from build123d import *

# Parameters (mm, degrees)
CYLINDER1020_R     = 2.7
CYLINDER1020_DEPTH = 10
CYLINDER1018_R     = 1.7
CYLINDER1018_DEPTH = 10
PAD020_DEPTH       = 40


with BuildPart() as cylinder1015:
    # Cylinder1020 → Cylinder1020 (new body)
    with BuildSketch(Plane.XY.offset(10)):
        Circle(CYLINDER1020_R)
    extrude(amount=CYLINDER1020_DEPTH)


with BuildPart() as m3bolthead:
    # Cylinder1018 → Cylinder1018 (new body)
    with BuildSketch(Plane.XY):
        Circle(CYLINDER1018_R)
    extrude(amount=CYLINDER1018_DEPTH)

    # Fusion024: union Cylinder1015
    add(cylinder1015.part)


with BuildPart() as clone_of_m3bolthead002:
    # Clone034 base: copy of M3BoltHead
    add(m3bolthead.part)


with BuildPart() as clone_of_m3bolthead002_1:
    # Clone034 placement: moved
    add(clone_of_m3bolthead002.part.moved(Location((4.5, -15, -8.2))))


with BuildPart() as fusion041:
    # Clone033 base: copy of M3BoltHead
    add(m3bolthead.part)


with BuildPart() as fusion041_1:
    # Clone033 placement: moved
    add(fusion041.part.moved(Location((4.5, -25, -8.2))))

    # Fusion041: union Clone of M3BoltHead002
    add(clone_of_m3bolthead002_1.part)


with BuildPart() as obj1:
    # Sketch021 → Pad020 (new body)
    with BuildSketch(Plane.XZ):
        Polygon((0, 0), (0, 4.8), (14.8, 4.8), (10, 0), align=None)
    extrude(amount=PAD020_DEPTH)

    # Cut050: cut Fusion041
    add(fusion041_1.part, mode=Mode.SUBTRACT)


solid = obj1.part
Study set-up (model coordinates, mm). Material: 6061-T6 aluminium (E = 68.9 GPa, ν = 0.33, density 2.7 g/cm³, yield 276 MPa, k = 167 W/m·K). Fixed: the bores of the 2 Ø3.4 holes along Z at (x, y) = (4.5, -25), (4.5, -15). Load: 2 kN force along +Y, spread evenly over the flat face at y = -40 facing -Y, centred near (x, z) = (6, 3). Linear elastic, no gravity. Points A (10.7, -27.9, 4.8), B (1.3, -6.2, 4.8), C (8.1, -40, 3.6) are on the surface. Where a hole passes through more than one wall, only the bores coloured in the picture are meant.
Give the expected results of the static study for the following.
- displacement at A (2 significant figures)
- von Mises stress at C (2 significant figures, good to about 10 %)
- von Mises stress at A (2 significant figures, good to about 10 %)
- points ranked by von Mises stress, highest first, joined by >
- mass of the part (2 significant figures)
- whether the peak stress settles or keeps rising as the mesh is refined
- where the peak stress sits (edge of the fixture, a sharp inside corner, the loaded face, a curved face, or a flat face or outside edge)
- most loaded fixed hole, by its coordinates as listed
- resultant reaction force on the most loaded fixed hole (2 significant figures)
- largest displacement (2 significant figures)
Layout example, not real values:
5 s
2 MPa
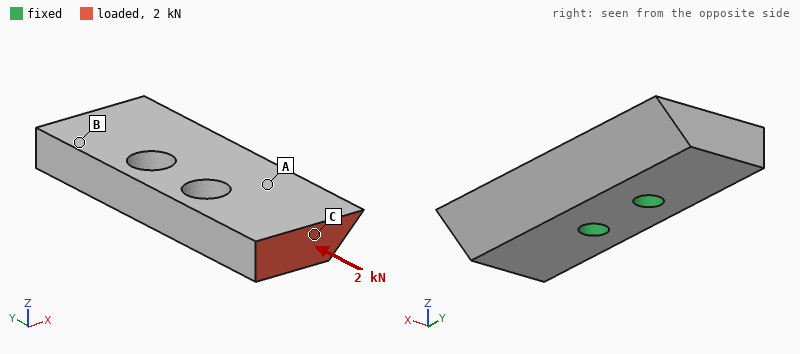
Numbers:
12 µm
33 MPa
53 MPa
A > C > B
6.0 g
keeps rising
edge of the fixture
(4.5, -25)
1.4 kN
31 µm
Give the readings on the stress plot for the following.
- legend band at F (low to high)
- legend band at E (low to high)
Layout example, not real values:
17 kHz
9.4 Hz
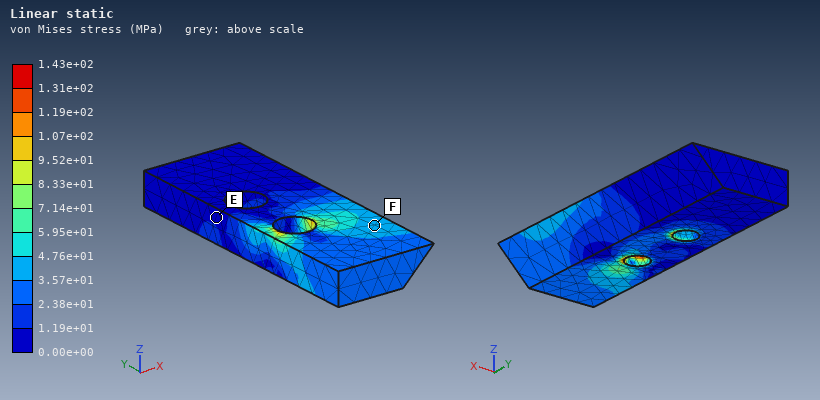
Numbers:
3.57e+01 to 4.76e+01 MPa
0.00e+00 to 1.19e+01 MPa
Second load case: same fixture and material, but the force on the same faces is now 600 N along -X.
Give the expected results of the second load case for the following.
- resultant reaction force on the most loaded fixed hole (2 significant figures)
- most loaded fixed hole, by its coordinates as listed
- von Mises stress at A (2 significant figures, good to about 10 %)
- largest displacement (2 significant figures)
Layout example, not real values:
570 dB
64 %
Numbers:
1.2 kN
(4.5, -25)
25 MPa
59 µm
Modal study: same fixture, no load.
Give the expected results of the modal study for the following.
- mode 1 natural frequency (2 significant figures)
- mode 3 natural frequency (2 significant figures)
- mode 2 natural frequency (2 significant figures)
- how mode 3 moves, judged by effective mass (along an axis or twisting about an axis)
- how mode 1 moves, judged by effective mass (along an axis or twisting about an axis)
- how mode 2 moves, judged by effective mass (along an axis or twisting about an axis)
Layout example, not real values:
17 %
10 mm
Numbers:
11 kHz
17 kHz
12 kHz
along X
twisting about X
along Z
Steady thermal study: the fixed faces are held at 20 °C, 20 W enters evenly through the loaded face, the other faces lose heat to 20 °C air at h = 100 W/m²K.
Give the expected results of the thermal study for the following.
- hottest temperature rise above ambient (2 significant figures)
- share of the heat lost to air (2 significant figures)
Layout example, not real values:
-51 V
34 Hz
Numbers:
35 K
6.5 %
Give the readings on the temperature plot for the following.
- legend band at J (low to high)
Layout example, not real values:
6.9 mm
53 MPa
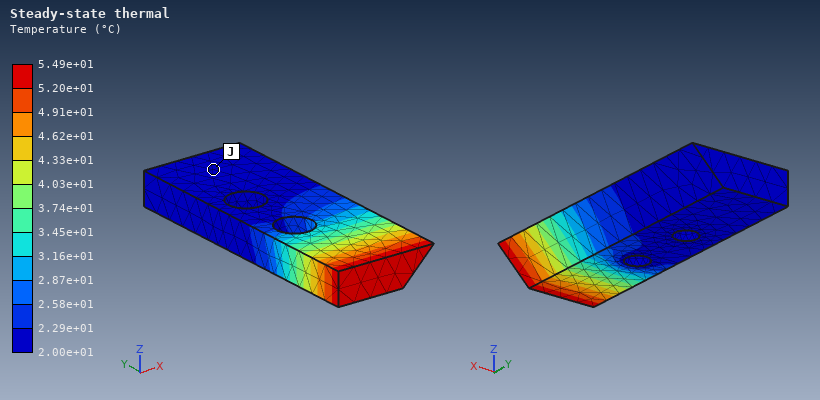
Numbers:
2.00e+01 to 2.29e+01 °C
